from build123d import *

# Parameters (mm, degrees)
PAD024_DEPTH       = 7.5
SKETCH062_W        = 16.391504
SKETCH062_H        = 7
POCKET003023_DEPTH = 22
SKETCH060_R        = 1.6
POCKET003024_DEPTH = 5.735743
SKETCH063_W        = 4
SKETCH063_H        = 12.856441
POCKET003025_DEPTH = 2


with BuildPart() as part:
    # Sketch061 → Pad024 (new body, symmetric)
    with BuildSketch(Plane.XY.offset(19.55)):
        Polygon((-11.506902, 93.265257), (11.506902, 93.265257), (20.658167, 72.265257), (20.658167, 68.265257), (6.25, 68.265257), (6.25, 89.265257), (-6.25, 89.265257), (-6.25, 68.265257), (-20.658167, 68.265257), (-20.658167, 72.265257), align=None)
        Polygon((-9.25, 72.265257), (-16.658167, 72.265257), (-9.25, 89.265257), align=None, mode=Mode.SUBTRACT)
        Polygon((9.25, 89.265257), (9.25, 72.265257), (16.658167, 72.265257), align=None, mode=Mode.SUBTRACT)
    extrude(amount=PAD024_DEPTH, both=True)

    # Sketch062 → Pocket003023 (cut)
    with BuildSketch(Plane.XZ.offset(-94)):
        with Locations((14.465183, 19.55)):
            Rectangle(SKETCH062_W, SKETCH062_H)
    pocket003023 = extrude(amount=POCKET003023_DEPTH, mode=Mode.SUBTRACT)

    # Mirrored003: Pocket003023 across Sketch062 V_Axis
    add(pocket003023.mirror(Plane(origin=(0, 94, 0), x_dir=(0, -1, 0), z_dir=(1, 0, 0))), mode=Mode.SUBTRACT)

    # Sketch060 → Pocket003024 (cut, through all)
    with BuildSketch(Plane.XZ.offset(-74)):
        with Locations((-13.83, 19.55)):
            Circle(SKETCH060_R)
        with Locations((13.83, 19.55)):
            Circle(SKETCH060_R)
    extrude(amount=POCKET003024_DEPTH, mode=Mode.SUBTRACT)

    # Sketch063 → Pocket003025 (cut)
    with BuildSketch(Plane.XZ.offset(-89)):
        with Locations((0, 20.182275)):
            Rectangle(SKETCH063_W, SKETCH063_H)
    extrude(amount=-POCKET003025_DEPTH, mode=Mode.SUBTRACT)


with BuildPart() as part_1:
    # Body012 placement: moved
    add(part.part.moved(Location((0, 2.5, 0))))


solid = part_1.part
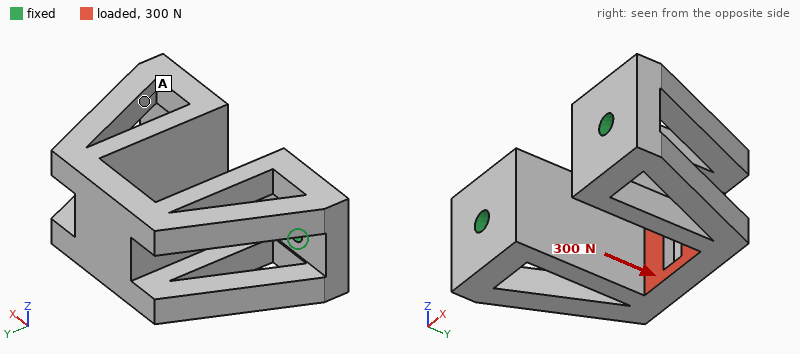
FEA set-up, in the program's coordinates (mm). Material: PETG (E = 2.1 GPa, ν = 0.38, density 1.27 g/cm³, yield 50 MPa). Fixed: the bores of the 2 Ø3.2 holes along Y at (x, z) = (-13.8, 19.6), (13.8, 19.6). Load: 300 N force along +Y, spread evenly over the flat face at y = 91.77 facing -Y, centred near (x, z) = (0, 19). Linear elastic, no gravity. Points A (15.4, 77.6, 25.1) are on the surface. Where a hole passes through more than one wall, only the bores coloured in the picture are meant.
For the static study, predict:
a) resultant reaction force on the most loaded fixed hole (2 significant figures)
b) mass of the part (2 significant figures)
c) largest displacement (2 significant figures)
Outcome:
160 N
5.8 g
0.21 mm
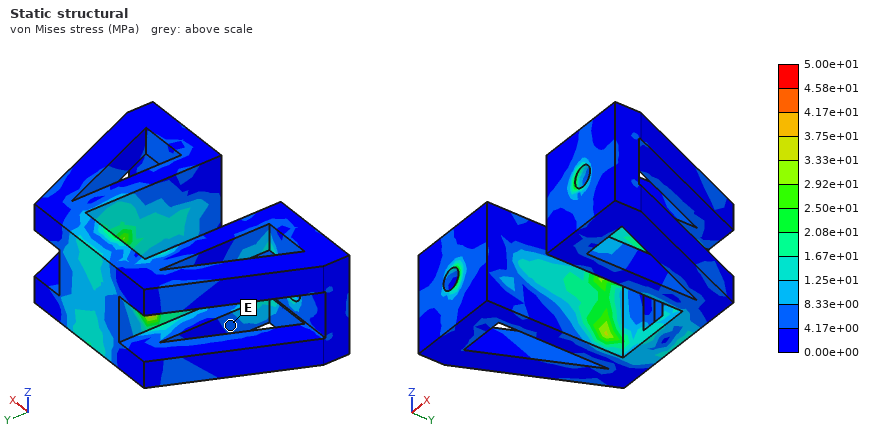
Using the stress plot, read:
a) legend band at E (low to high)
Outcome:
4.17e+00 to 8.33e+00 MPa
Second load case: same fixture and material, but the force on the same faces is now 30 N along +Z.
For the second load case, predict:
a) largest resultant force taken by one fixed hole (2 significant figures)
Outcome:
15 N
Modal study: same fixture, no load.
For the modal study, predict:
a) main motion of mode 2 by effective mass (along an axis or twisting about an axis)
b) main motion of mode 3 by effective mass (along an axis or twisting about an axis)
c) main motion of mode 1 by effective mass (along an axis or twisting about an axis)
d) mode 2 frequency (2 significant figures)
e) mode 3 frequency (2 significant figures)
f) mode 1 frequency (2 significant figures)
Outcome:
along X
twisting about Y
along Z
1800 Hz
2200 Hz
1200 Hz
